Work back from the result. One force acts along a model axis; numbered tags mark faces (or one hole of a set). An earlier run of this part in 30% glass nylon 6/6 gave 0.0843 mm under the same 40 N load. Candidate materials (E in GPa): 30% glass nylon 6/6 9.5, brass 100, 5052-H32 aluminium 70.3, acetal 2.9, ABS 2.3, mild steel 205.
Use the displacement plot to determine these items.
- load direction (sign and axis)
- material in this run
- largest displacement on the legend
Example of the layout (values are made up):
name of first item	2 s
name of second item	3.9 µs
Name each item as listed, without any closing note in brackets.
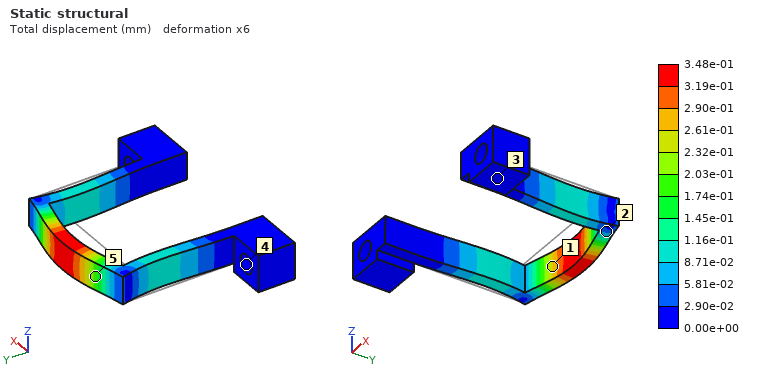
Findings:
load direction	+Y
material in this run	ABS
largest displacement on the legend	3.48e-01 mm
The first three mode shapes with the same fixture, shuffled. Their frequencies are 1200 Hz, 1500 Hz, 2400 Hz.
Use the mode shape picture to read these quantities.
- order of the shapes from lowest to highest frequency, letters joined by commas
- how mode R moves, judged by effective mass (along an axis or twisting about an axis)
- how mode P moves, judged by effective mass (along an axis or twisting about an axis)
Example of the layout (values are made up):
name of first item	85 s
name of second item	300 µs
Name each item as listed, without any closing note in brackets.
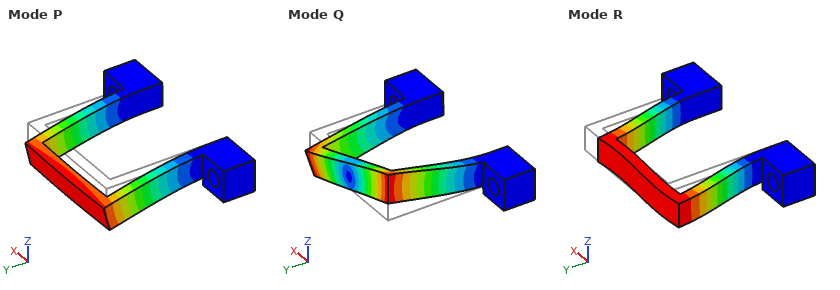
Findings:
order of the shapes from lowest to highest frequency, letters joined by commas	R, P, Q
how mode R moves, judged by effective mass	along X
how mode P moves, judged by effective mass	along Z
